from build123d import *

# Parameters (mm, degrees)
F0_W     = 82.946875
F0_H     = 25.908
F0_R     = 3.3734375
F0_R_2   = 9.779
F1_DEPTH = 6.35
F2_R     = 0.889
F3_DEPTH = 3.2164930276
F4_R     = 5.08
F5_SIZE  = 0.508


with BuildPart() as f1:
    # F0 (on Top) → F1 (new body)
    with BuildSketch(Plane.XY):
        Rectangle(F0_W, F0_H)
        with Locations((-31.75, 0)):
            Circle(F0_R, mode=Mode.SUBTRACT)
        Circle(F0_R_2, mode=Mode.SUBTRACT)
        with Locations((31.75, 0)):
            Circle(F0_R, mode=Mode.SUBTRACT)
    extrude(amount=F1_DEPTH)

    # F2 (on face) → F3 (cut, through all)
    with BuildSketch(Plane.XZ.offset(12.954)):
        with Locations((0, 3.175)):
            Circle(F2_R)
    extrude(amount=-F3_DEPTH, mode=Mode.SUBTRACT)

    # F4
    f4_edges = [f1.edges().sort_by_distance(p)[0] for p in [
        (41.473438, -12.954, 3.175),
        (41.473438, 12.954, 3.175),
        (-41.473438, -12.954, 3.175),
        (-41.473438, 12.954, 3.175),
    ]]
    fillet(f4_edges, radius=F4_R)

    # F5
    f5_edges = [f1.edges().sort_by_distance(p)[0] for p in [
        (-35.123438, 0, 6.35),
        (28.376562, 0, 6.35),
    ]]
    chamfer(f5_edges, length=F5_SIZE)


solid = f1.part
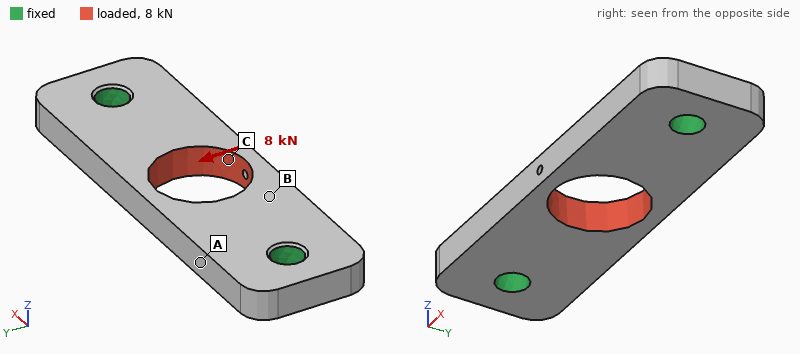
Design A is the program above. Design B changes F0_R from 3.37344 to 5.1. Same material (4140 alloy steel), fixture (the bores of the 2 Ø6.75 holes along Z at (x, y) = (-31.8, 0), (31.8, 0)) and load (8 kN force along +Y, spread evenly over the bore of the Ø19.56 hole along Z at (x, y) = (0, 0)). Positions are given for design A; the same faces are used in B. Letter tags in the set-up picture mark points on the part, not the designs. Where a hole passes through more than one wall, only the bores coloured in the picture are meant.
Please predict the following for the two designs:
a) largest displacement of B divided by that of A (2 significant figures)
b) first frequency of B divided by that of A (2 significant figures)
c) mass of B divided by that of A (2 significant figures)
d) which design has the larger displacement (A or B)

0.81
1.2
0.95
A
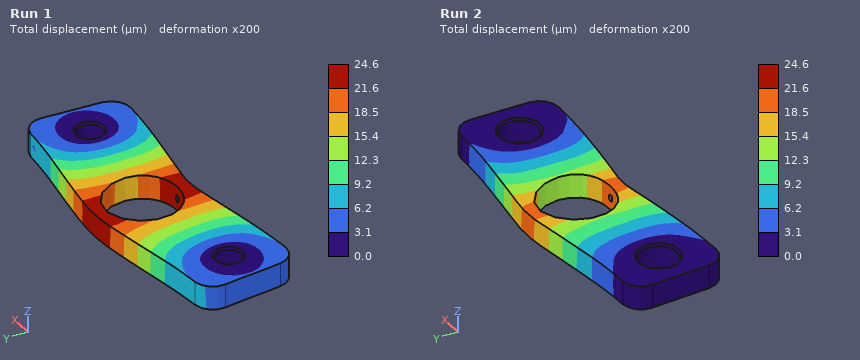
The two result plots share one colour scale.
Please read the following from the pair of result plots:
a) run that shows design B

Run 2
